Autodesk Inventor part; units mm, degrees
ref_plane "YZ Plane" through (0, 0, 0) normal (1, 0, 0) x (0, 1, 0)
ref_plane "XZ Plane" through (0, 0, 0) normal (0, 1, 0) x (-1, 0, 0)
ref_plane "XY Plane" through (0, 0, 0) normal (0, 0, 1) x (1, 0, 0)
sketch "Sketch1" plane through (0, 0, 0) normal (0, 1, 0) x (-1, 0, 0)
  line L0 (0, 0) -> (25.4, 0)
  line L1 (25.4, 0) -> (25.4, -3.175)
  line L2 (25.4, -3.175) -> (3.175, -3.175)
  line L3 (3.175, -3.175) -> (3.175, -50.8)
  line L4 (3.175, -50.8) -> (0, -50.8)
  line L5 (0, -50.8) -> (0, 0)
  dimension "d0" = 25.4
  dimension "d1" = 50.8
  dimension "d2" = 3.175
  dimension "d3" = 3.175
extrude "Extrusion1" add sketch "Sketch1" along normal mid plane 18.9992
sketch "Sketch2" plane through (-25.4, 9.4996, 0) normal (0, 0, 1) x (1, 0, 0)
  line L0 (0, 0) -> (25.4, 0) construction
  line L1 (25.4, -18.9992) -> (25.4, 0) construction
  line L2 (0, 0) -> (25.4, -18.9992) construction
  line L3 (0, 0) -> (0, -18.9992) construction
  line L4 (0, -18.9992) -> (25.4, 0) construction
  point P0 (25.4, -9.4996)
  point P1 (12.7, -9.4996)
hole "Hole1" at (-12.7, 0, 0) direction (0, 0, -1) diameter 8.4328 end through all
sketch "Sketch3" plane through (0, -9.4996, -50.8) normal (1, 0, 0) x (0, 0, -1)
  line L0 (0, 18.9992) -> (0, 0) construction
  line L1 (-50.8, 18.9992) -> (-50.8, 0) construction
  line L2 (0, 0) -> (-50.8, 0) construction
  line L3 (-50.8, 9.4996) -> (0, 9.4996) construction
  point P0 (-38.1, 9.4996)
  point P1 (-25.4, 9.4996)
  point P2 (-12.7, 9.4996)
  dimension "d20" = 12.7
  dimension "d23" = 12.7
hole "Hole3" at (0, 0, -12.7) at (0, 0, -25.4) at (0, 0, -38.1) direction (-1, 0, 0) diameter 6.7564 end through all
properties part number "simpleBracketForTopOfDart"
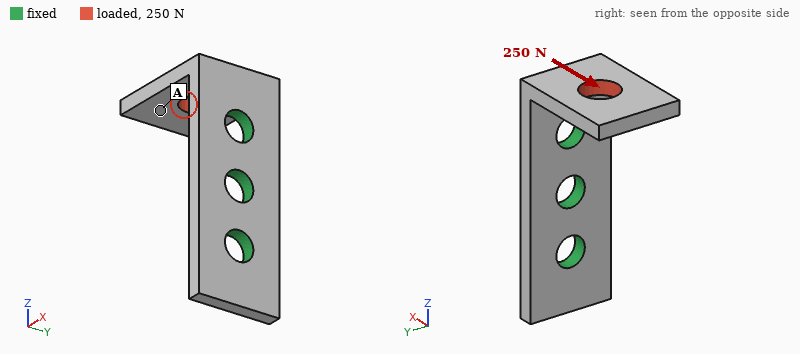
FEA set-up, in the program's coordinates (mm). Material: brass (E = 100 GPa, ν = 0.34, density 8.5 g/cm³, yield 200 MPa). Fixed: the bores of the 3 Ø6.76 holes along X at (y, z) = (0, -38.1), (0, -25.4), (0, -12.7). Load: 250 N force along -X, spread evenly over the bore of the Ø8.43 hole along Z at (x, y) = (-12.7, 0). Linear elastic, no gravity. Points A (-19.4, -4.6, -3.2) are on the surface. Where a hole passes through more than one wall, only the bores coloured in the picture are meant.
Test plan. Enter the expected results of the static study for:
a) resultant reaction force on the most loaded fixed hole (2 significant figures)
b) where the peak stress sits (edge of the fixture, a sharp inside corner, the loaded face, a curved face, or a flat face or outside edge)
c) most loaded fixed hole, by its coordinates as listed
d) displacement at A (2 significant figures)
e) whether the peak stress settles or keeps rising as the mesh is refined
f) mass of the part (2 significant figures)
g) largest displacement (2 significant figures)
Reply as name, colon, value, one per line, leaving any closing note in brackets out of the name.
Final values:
resultant reaction force on the most loaded fixed hole: 270 N
where the peak stress sits: edge of the fixture
most loaded fixed hole, by its coordinates as listed: (0, -12.7)
displacement at A: 37 µm
whether the peak stress settles or keeps rising as the mesh is refined: keeps rising
mass of the part: 33 g
largest displacement: 50 µm
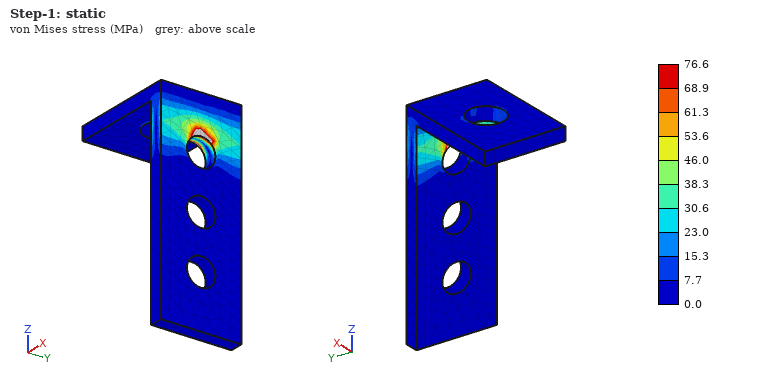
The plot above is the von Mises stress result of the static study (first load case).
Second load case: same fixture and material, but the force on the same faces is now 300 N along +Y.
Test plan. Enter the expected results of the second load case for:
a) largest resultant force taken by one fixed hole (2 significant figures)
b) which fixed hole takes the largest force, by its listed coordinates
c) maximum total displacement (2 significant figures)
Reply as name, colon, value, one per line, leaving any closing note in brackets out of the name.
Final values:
largest resultant force taken by one fixed hole: 380 N
which fixed hole takes the largest force, by its listed coordinates: (0, -12.7)
maximum total displacement: 79 µm
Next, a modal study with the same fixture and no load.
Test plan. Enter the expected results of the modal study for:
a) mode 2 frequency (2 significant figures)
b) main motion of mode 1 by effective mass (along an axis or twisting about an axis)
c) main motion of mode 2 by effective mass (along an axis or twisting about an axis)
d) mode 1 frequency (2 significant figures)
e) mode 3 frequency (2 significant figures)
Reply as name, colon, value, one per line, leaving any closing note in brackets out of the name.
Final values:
mode 2 frequency: 3300 Hz
main motion of mode 1 by effective mass: along Z
main motion of mode 2 by effective mass: along Y
mode 1 frequency: 2000 Hz
mode 3 frequency: 7000 Hz
